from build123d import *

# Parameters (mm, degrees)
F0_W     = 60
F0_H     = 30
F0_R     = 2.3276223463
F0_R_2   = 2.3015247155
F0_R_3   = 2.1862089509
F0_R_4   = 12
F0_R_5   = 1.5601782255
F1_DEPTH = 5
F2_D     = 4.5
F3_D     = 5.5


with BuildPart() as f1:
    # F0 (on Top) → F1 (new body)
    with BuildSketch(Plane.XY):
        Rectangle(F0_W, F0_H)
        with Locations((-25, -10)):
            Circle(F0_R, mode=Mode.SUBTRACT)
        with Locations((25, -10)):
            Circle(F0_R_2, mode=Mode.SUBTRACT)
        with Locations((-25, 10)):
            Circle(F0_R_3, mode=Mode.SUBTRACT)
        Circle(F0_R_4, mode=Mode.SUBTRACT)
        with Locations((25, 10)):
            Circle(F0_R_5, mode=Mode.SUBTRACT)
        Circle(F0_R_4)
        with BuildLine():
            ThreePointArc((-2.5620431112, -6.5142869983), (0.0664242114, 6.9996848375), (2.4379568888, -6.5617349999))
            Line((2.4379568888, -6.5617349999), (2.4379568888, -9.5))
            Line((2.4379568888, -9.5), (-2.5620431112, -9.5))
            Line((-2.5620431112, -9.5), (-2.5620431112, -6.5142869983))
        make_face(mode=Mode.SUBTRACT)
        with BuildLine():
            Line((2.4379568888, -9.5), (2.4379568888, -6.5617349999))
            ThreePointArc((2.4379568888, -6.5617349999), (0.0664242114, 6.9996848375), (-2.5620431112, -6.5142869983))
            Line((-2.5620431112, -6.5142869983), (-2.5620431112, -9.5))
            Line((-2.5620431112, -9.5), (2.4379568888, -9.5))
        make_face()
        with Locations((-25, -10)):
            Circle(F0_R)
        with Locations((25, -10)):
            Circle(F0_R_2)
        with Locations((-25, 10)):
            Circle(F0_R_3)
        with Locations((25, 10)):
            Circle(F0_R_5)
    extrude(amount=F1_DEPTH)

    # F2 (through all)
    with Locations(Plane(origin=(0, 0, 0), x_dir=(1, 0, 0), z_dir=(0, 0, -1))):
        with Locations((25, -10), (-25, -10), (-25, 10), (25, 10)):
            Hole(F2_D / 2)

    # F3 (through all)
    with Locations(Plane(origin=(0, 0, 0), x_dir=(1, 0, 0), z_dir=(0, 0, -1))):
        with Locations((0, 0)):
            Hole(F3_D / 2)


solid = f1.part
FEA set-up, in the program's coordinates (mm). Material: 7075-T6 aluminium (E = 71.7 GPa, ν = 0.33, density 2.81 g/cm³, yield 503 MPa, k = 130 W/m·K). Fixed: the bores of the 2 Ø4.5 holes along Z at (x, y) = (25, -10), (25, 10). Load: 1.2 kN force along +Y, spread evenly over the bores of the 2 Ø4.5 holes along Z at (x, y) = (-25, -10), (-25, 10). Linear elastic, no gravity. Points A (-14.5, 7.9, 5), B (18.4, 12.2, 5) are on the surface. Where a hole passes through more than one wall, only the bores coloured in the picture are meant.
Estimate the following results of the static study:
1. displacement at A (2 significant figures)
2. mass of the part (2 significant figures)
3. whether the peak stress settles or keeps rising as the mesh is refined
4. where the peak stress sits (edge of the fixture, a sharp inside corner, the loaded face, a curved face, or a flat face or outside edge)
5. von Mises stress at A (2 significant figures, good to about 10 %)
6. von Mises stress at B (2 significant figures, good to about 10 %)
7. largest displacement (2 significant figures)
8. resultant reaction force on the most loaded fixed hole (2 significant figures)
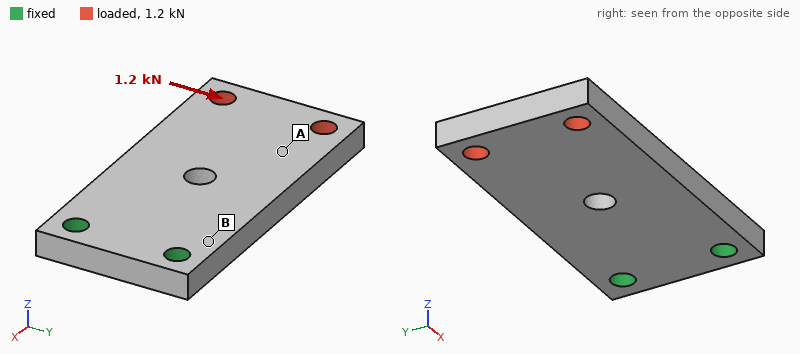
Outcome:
59 µm
24 g
keeps rising
edge of the fixture
18 MPa
58 MPa
94 µm
2.8 kN
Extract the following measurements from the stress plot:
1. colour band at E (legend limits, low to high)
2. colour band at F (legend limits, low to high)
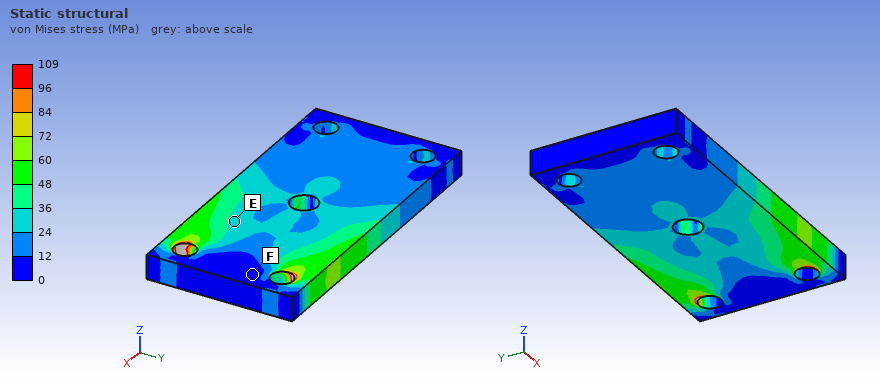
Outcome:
24 to 36 MPa
0 to 12 MPa
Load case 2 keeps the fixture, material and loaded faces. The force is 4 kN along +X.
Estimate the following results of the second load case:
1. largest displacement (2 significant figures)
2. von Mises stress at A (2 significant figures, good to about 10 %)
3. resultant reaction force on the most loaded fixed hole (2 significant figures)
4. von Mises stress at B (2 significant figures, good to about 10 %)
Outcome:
25 µm
26 MPa
2.0 kN
33 MPa
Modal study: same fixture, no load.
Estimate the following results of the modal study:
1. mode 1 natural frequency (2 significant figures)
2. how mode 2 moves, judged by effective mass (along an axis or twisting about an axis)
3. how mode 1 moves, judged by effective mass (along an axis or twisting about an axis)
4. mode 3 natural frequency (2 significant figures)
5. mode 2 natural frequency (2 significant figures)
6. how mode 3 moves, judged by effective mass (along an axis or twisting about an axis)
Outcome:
1400 Hz
twisting about X
along Z
6900 Hz
5200 Hz
along Y
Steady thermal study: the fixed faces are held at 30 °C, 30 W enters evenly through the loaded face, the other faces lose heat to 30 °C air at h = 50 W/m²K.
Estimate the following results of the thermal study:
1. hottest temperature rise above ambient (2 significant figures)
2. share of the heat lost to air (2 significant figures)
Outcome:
72 K
24 %
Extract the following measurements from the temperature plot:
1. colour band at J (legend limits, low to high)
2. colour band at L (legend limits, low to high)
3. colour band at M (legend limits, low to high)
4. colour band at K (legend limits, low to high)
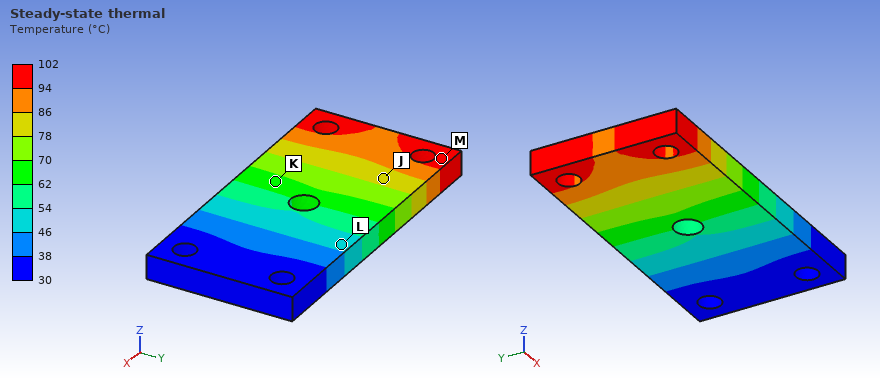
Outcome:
78 to 86 °C
46 to 54 °C
94 to 102 °C
62 to 70 °C
